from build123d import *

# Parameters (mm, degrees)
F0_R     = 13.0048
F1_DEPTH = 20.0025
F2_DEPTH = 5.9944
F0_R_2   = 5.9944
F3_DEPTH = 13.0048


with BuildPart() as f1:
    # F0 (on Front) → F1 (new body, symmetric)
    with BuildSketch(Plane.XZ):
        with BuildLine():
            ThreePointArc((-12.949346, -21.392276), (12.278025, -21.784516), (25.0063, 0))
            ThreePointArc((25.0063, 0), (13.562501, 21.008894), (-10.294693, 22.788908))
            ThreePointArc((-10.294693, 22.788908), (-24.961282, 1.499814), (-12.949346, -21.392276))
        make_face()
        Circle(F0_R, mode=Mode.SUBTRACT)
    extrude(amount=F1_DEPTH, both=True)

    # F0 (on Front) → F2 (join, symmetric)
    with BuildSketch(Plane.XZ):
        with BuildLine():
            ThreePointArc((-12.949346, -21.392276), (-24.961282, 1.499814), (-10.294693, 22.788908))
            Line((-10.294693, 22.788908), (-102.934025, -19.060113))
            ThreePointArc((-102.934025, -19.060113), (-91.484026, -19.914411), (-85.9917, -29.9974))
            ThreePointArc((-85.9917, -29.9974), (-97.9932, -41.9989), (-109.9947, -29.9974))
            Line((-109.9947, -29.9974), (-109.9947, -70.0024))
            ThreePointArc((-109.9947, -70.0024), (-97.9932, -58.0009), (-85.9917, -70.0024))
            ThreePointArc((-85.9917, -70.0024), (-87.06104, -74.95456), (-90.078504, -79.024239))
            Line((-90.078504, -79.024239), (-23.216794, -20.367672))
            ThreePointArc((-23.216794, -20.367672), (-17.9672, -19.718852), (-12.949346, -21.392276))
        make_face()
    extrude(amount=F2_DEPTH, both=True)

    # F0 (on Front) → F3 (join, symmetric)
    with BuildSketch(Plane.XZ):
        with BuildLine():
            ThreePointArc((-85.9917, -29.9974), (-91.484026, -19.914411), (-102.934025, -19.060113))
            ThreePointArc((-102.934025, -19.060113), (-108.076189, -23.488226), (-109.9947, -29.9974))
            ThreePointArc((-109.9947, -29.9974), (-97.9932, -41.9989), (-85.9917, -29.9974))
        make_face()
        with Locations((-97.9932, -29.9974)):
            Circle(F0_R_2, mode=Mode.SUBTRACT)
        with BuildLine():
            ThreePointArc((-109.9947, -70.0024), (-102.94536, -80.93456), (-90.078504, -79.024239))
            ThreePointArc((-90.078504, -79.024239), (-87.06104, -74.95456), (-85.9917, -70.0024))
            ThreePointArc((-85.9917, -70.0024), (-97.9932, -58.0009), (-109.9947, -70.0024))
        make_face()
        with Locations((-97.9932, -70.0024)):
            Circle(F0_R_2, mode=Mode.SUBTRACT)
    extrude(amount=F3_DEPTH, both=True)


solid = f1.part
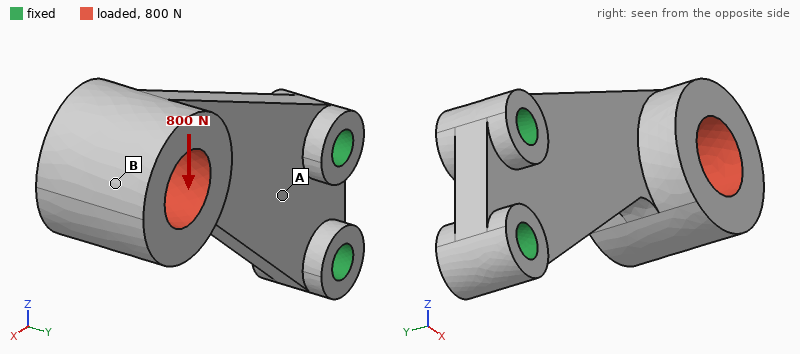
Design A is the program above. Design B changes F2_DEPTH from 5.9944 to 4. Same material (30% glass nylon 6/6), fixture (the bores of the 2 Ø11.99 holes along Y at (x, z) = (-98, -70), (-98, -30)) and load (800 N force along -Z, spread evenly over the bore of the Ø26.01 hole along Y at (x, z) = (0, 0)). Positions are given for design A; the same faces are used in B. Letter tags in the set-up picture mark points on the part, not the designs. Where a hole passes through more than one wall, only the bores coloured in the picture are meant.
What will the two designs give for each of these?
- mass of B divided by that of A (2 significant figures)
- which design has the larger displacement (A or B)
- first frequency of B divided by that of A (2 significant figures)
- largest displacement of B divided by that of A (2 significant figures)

0.87
B
0.57
1.5
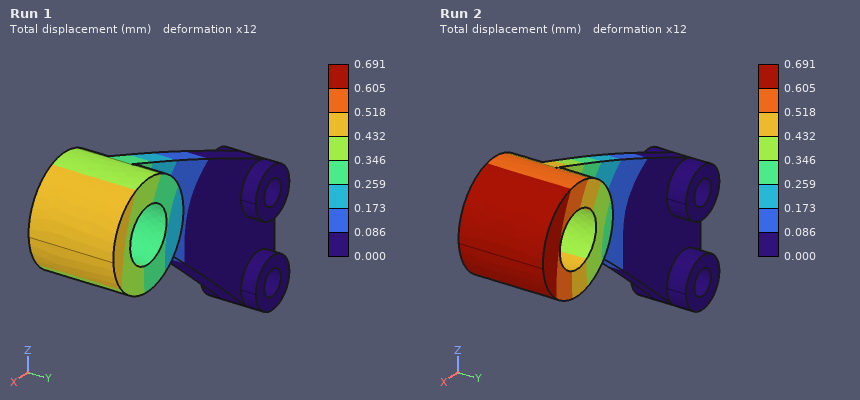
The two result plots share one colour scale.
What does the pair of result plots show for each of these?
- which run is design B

Run 2
